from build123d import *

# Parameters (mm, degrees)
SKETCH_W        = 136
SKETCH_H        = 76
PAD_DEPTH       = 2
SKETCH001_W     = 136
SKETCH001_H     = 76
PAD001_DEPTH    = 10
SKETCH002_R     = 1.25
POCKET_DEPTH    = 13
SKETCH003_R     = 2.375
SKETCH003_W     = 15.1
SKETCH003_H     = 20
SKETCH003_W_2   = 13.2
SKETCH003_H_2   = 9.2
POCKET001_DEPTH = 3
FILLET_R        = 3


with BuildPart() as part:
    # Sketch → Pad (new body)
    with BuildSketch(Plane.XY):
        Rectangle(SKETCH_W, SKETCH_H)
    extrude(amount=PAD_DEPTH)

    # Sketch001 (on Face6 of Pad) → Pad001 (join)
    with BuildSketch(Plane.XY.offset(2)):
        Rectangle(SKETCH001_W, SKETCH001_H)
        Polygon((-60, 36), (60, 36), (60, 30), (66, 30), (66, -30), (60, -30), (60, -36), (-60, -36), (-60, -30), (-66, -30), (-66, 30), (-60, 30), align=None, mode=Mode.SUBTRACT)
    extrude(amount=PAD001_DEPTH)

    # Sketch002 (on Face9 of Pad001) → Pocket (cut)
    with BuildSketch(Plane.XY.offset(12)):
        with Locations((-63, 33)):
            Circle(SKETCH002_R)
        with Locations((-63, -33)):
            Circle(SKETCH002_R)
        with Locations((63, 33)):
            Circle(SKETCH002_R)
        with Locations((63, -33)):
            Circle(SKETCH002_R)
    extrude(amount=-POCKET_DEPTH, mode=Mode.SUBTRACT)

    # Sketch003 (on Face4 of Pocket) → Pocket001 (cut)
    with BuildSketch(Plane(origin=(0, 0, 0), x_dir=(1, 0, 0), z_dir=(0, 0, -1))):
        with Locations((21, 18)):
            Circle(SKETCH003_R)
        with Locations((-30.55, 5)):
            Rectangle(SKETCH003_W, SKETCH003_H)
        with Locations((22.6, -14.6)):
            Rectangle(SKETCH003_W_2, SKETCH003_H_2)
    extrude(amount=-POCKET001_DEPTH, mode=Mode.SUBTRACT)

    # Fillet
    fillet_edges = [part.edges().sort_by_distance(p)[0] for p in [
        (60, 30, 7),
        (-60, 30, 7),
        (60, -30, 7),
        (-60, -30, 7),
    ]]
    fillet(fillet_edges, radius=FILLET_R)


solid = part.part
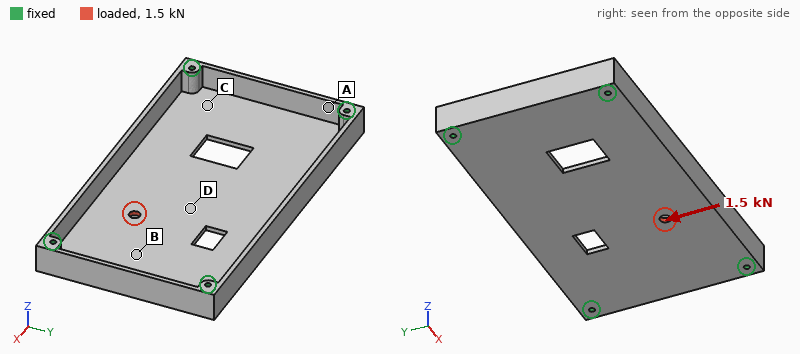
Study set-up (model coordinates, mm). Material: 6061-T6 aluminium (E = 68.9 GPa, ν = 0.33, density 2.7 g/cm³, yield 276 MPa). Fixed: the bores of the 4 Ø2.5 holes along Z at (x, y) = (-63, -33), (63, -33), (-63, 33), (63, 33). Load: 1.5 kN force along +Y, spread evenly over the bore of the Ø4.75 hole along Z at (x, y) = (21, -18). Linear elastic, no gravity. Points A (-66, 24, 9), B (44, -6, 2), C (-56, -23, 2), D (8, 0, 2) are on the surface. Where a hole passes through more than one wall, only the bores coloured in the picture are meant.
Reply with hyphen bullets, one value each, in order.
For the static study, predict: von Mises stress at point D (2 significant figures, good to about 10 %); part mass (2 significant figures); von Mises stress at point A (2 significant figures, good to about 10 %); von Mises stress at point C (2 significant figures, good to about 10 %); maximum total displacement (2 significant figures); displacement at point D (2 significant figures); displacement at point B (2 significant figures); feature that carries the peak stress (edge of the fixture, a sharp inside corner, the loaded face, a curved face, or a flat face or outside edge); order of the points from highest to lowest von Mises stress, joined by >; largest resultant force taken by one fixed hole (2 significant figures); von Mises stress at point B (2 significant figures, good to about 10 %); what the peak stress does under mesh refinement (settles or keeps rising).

- 11 MPa
- 79 g
- 3.0 MPa
- 5.9 MPa
- 30 µm
- 17 µm
- 9.1 µm
- a sharp inside corner
- B > D > C > A
- 670 N
- 16 MPa
- keeps rising
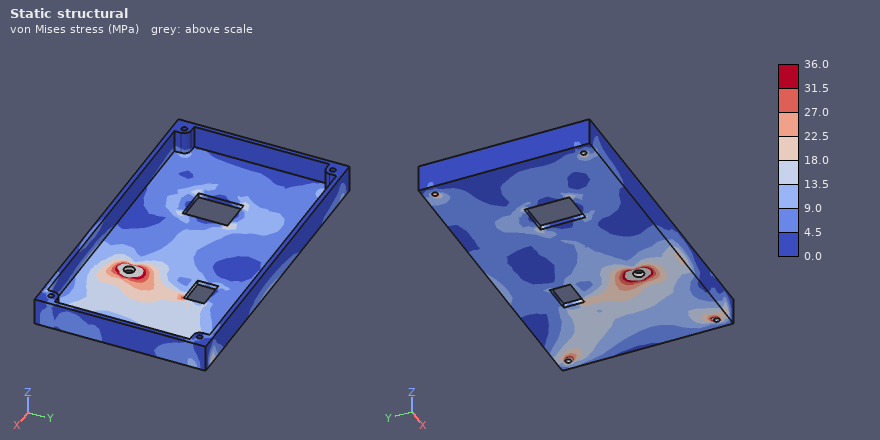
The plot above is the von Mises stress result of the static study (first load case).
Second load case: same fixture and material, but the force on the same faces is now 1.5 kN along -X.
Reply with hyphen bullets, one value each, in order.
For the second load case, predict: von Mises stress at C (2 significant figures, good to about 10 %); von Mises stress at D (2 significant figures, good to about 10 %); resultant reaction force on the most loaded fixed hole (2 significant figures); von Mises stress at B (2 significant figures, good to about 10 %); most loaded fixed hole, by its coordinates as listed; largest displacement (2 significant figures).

- 4.3 MPa
- 5.6 MPa
- 660 N
- 4.9 MPa
- (63, -33)
- 13 µm
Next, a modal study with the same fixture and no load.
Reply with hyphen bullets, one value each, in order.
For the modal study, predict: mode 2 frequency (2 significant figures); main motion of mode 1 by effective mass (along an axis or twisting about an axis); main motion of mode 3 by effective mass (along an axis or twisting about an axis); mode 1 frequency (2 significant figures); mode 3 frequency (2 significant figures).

- 2300 Hz
- along Z
- twisting about X
- 1200 Hz
- 2800 Hz
